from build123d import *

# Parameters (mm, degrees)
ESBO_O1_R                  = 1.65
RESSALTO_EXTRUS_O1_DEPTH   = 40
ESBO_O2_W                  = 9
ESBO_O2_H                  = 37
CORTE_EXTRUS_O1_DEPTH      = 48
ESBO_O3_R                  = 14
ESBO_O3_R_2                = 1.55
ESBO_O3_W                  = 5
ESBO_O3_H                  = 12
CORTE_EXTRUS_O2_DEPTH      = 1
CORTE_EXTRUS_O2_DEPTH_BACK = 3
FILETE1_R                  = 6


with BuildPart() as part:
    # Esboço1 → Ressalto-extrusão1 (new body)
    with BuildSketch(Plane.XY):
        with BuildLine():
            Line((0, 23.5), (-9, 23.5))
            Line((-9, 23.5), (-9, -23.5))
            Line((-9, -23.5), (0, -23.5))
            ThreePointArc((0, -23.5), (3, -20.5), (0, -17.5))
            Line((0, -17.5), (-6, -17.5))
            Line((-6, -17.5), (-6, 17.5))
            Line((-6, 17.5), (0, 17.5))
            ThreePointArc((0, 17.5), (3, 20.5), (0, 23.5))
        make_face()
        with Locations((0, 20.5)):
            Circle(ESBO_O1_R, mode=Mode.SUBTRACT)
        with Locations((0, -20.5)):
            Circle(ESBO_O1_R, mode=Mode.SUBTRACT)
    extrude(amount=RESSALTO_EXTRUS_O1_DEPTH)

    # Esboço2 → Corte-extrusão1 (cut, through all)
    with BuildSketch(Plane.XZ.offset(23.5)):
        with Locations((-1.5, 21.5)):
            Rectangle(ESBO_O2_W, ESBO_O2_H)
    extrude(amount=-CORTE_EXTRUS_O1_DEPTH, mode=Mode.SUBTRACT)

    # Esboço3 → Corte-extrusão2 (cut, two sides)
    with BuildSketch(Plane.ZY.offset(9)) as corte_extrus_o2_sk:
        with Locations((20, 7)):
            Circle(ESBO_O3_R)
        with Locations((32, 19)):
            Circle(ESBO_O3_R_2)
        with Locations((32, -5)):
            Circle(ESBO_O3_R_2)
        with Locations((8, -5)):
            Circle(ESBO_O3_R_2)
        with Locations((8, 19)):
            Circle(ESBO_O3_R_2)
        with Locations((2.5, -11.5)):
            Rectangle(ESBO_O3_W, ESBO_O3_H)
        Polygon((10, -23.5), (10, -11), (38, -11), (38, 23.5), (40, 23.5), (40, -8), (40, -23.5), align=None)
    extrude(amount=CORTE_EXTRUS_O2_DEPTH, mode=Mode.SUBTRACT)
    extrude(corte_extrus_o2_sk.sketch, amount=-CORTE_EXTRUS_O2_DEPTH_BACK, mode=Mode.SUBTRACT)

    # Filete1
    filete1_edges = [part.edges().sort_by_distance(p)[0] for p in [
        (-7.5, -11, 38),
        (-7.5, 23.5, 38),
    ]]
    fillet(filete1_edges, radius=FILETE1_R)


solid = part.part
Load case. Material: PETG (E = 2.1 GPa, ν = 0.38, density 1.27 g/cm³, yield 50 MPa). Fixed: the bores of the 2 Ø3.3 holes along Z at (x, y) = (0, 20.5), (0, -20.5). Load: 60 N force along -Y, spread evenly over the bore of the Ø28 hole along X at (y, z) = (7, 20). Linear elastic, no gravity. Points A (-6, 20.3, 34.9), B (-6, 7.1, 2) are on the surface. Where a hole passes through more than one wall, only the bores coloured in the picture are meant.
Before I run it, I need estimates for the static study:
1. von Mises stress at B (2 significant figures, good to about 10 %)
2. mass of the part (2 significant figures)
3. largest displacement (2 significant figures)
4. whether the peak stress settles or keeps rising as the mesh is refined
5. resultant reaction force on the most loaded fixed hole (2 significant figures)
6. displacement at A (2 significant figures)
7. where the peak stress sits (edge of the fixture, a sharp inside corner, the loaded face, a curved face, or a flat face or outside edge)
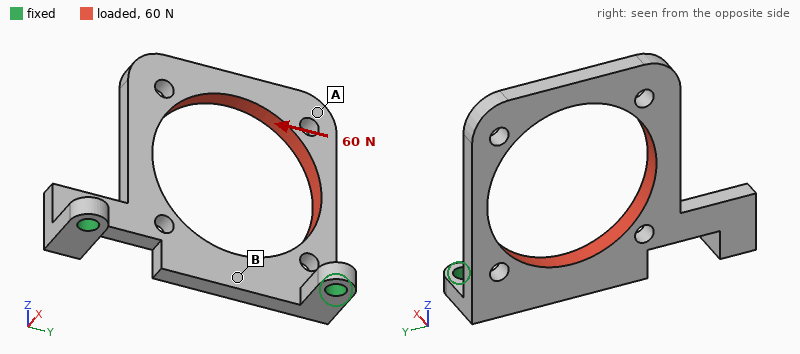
4.9 MPa
3.0 g
0.66 mm
keeps rising
40 N
0.65 mm
edge of the fixture
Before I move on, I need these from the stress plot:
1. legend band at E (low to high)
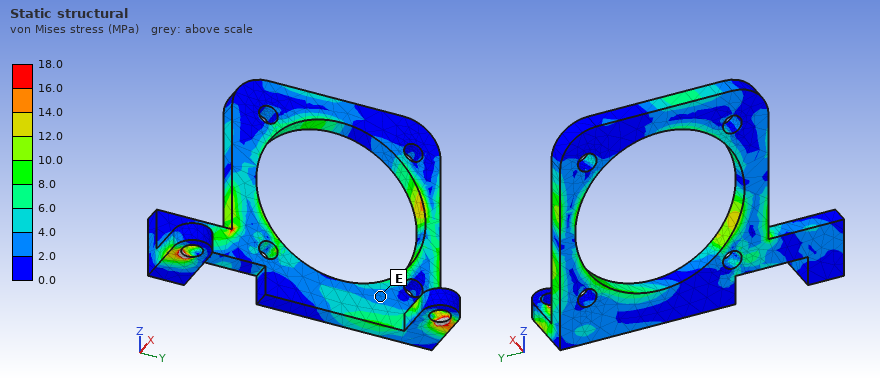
2.0 to 4.0 MPa
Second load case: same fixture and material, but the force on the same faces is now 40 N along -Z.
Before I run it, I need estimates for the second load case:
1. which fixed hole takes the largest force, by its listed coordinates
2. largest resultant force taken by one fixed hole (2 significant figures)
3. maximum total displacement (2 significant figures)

(0, 20.5)
28 N
0.62 mm
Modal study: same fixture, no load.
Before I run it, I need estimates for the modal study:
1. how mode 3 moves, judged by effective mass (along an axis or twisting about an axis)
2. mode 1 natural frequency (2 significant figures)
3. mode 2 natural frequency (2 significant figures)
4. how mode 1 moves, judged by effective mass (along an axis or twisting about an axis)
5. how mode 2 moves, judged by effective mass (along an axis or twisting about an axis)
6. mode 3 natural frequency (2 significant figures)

along Y
260 Hz
760 Hz
along X
twisting about Z
1200 Hz
